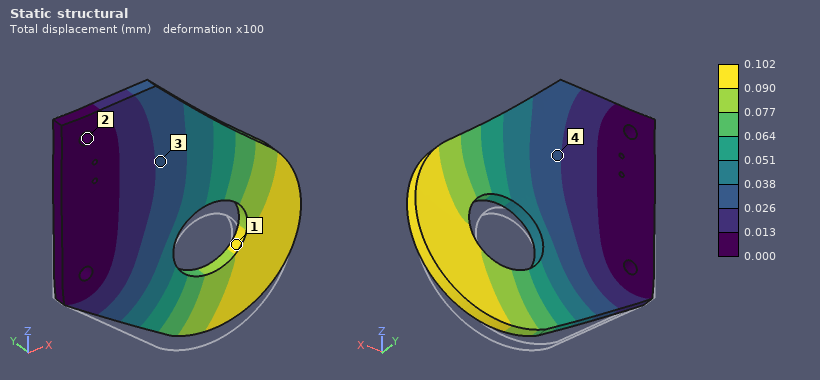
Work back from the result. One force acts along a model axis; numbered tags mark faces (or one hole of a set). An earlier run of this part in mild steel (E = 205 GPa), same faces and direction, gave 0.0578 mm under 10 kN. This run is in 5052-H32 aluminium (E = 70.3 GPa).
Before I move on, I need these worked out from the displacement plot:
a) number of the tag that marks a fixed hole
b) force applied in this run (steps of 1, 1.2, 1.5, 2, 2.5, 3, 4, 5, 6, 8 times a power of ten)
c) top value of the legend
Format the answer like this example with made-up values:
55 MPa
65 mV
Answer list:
2
6 kN
0.102 mm
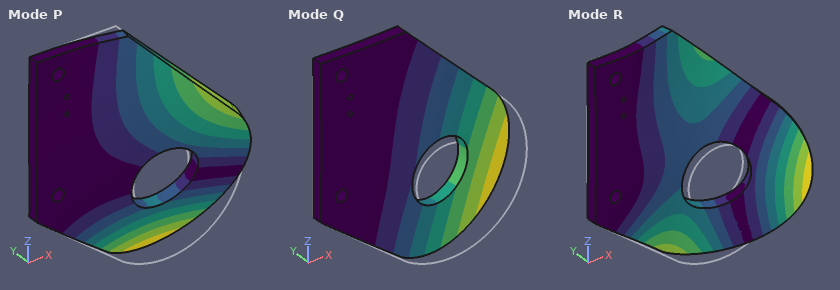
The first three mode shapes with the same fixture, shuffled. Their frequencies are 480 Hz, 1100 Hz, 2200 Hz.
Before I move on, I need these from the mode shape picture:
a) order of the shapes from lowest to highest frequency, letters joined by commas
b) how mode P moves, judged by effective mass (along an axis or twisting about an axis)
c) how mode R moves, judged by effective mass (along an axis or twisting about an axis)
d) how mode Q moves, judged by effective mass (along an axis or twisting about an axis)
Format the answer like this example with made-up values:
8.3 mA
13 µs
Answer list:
Q, P, R
twisting about X
along Y
along Y
